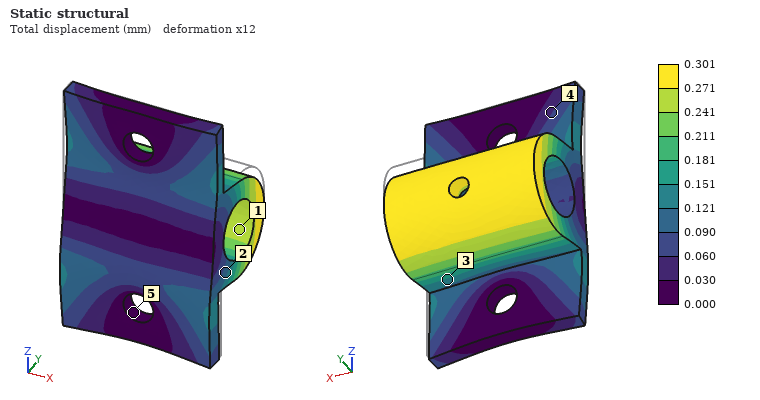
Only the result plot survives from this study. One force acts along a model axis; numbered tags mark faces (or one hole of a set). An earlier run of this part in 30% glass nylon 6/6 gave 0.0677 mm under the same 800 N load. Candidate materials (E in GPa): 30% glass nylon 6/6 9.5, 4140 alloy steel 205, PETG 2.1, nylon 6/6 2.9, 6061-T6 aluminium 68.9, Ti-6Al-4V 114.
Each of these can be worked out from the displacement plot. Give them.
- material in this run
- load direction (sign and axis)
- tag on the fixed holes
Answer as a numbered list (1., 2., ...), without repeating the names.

1. PETG
2. -Z
3. 5
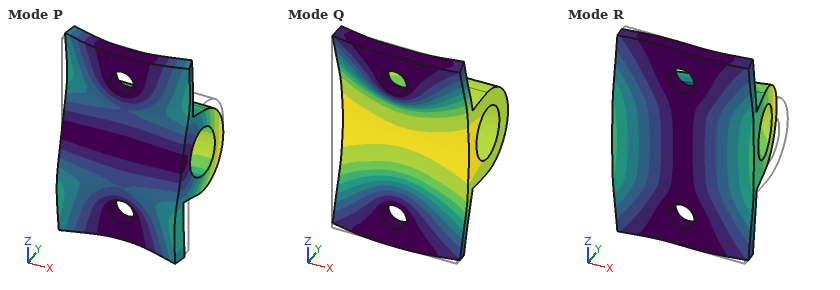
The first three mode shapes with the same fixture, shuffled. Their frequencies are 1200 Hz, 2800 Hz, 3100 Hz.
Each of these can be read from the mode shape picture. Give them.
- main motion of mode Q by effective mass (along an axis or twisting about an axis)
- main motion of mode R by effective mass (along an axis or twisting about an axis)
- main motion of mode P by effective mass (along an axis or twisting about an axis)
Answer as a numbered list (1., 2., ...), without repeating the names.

1. along Y
2. along X
3. along Z
